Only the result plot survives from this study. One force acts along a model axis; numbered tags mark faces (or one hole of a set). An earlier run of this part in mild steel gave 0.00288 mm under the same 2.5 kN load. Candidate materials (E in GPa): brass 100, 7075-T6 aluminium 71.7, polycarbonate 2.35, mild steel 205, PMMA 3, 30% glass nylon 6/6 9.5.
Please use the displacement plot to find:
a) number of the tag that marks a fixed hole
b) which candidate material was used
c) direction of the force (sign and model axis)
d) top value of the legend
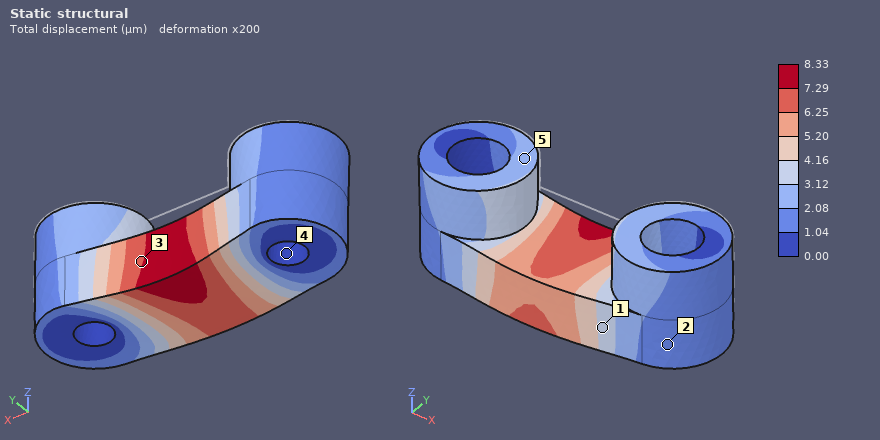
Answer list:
4
7075-T6 aluminium
-Y
8.33 µm
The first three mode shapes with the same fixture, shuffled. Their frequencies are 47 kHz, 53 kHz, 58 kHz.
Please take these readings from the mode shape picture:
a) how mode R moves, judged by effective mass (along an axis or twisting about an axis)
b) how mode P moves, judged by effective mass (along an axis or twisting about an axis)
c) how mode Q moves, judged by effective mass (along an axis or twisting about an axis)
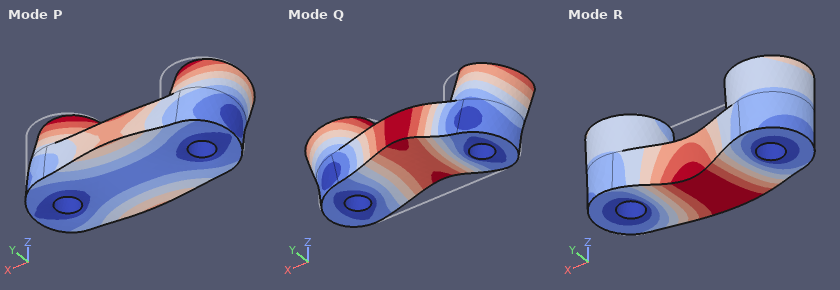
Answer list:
along Y
along Y
along Z
